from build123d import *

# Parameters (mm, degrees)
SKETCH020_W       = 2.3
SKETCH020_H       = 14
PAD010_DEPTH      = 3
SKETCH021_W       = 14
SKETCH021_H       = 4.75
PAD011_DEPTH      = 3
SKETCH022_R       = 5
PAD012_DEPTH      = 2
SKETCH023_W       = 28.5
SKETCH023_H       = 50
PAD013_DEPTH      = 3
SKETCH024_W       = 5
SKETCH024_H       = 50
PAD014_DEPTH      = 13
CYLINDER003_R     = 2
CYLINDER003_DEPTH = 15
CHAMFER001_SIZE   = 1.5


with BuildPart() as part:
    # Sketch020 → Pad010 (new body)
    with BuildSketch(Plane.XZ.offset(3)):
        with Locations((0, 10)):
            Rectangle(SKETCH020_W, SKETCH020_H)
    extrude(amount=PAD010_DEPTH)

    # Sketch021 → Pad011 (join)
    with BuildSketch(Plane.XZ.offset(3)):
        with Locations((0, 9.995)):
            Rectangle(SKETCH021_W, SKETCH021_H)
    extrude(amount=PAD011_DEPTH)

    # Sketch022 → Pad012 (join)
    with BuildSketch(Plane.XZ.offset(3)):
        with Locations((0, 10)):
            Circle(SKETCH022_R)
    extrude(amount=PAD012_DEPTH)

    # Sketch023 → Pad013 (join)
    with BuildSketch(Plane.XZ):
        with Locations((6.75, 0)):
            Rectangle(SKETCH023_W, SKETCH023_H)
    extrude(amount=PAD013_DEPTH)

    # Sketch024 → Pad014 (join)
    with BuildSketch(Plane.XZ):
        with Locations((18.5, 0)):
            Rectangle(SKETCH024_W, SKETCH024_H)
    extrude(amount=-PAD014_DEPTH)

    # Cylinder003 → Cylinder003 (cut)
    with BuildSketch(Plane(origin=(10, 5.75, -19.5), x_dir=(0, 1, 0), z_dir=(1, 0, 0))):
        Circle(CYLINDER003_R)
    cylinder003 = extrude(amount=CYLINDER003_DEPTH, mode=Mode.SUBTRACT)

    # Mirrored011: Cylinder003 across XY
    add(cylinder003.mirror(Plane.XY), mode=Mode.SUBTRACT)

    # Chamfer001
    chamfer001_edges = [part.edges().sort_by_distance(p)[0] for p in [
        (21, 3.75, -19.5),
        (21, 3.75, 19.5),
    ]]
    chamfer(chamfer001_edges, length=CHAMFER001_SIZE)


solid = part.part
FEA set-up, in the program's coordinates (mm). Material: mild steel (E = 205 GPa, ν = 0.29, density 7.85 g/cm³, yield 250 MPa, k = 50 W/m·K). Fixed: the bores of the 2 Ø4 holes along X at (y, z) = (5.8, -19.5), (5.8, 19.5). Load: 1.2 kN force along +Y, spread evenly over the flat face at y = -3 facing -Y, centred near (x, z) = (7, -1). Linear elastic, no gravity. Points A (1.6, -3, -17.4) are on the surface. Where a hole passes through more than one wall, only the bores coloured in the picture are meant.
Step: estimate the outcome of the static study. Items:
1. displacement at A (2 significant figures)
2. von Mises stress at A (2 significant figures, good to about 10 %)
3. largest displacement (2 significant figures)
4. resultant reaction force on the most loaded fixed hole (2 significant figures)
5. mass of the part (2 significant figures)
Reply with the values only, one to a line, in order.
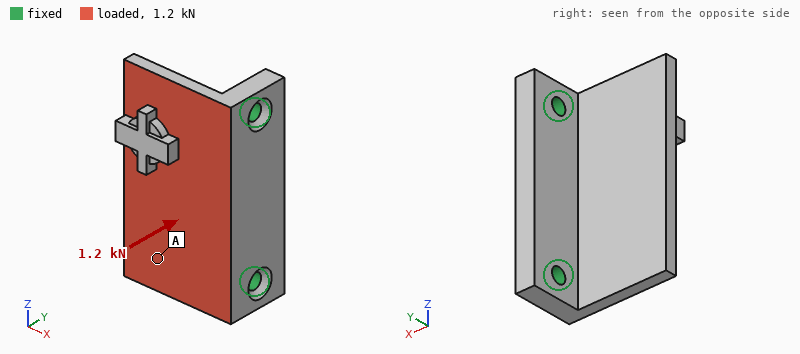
0.070 mm
22 MPa
0.12 mm
630 N
60 g
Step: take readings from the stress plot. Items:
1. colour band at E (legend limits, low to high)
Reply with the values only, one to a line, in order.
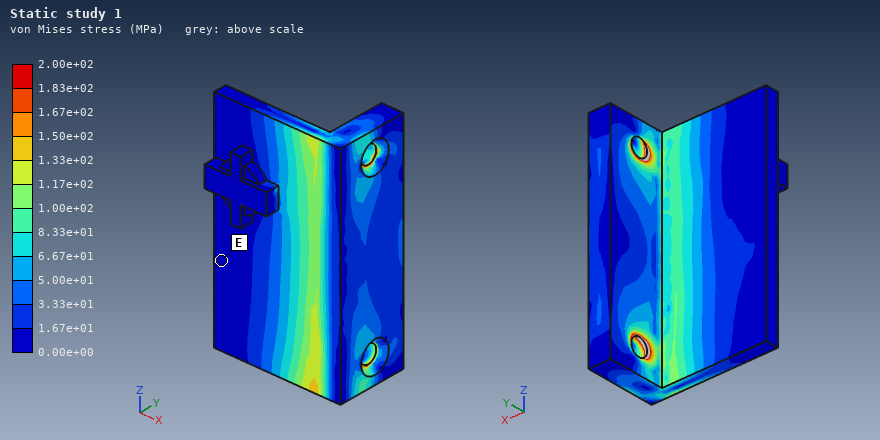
0.00e+00 to 1.67e+01 MPa
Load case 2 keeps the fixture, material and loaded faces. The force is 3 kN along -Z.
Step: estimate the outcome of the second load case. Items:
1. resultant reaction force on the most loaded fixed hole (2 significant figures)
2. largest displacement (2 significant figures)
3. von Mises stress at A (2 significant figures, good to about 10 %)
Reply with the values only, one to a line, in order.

1.8 kN
15 µm
20 MPa
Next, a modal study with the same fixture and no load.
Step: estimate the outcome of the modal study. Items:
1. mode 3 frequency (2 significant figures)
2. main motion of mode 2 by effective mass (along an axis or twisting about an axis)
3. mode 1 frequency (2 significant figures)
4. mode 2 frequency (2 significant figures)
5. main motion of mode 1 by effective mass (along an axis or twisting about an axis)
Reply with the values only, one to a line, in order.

11 kHz
twisting about X
3100 Hz
5700 Hz
along Y
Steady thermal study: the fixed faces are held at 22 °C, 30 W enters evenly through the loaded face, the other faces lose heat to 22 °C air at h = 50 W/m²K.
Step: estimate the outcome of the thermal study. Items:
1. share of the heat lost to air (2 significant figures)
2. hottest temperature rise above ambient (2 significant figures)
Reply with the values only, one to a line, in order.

18 %
61 K
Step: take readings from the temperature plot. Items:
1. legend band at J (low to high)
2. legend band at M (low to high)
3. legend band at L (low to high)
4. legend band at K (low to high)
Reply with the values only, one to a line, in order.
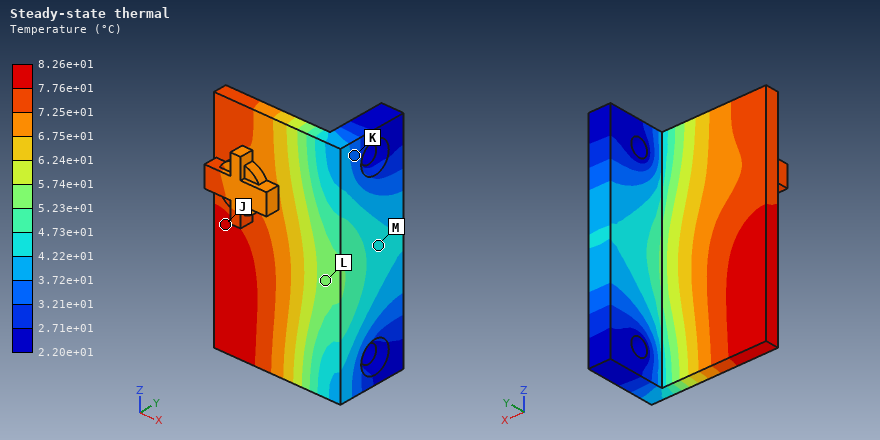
7.76e+01 to 8.26e+01 °C
4.22e+01 to 4.73e+01 °C
5.23e+01 to 5.74e+01 °C
3.21e+01 to 3.72e+01 °C
